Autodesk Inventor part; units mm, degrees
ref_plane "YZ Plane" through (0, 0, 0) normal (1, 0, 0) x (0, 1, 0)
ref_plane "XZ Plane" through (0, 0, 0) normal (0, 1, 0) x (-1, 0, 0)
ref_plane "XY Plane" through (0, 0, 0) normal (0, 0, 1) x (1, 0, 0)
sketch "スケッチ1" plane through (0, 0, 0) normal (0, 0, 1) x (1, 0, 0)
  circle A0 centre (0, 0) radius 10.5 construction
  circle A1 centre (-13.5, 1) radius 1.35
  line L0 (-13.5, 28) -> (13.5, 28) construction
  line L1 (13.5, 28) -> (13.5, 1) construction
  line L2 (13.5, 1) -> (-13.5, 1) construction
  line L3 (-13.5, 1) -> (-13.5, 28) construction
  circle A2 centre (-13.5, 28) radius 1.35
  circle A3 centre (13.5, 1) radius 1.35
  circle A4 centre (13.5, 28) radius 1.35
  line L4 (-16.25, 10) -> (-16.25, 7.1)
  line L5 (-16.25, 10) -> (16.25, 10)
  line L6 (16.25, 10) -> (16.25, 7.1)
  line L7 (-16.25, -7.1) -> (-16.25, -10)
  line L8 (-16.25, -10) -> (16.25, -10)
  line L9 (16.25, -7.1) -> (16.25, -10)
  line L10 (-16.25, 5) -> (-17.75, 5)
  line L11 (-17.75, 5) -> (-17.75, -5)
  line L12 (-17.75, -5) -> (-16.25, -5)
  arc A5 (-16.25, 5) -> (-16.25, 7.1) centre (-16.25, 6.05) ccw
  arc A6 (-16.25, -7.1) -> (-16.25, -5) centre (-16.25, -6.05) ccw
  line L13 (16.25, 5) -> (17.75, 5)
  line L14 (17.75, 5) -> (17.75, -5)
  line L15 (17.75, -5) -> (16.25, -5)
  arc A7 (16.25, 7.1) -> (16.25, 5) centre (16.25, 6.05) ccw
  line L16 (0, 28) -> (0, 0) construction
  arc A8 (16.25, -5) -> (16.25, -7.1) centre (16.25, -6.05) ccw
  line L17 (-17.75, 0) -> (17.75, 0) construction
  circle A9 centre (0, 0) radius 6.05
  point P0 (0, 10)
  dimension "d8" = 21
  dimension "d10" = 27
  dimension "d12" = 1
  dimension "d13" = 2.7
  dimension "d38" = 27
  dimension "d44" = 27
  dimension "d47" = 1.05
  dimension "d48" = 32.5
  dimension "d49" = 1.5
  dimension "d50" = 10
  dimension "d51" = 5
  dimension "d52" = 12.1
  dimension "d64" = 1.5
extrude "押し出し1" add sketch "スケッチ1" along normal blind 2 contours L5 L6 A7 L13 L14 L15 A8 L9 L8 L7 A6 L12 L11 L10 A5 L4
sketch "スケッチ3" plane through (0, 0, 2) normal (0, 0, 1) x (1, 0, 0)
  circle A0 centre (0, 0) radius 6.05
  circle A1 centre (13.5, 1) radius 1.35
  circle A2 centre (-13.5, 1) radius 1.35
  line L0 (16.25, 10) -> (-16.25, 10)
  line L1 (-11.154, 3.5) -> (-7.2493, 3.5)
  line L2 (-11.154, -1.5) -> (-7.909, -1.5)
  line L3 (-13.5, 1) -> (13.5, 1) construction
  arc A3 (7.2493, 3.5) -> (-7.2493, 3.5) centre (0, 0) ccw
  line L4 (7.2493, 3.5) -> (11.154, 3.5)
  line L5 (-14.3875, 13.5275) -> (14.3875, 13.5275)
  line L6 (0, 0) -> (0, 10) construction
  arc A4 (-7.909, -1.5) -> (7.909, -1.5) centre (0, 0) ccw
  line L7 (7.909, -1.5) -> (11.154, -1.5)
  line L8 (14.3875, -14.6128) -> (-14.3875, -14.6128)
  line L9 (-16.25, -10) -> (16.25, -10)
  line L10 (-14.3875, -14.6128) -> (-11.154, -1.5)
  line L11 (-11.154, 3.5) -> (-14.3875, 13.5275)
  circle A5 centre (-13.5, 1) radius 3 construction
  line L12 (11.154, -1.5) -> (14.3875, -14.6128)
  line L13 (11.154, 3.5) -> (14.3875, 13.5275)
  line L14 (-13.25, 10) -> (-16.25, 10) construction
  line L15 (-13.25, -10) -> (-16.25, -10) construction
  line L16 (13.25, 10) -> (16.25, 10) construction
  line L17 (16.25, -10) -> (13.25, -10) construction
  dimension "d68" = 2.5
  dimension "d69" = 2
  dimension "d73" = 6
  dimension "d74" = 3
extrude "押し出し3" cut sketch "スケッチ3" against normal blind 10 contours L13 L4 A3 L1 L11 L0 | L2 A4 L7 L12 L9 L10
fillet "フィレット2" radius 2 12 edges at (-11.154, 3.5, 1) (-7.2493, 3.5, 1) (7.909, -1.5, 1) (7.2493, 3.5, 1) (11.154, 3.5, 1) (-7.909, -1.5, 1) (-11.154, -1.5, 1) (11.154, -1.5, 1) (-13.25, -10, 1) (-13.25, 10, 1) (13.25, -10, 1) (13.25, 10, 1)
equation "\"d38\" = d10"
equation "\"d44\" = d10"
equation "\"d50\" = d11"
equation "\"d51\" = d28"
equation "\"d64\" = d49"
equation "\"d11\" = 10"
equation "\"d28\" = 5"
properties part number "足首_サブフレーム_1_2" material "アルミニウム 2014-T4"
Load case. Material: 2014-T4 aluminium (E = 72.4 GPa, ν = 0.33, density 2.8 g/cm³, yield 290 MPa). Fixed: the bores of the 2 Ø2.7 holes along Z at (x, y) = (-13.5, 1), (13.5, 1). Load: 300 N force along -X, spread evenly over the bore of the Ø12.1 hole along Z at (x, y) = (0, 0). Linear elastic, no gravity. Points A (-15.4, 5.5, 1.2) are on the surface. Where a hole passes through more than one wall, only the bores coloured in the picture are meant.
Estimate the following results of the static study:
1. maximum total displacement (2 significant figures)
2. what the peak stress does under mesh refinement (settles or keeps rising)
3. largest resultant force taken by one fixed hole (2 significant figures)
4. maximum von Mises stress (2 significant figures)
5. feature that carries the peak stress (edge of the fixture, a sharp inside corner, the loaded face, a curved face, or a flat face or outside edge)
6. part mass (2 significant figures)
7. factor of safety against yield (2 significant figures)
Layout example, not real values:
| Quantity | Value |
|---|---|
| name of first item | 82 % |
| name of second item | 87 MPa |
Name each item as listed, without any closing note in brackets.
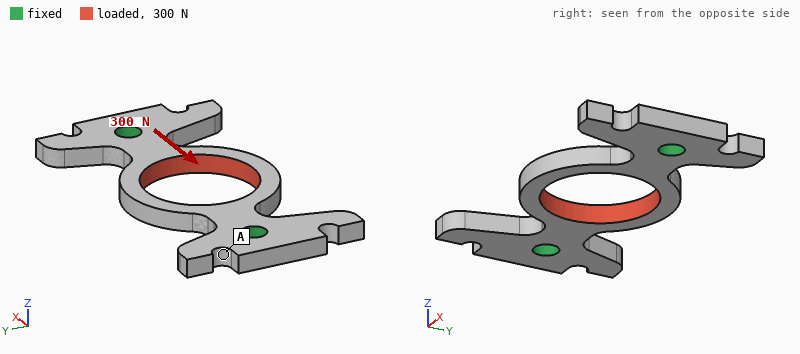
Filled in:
| Quantity | Value |
|---|---|
| maximum total displacement | 9.8 µm |
| what the peak stress does under mesh refinement | settles |
| largest resultant force taken by one fixed hole | 150 N |
| maximum von Mises stress | 75 MPa |
| feature that carries the peak stress | a curved face |
| part mass | 1.7 g |
| factor of safety against yield | 3.9 |
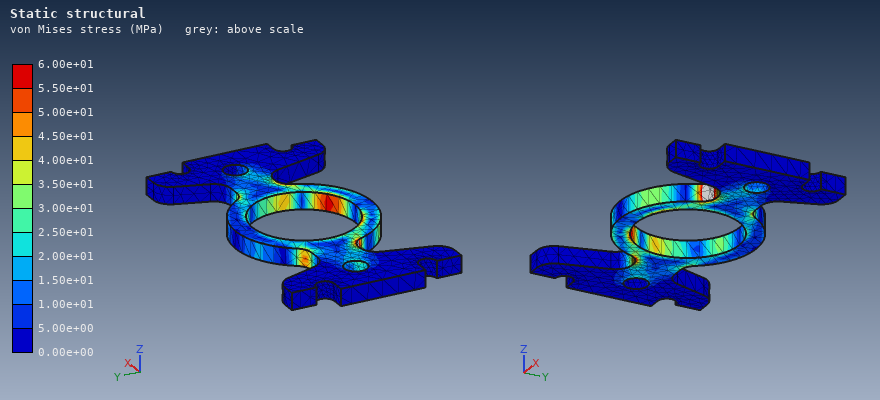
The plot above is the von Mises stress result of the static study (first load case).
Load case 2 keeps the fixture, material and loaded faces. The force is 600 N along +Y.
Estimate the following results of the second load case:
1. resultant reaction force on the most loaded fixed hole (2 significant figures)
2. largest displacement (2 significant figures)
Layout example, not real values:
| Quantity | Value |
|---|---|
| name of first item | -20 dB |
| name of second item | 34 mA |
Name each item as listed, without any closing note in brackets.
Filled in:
| Quantity | Value |
|---|---|
| resultant reaction force on the most loaded fixed hole | 300 N |
| largest displacement | 16 µm |
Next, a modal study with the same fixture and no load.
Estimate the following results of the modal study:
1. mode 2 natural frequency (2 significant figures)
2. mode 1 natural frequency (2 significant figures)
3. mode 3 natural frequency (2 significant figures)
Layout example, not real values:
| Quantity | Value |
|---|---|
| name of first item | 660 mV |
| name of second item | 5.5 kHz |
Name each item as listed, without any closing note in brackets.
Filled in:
| Quantity | Value |
|---|---|
| mode 2 natural frequency | 14 kHz |
| mode 1 natural frequency | 11 kHz |
| mode 3 natural frequency | 21 kHz |
